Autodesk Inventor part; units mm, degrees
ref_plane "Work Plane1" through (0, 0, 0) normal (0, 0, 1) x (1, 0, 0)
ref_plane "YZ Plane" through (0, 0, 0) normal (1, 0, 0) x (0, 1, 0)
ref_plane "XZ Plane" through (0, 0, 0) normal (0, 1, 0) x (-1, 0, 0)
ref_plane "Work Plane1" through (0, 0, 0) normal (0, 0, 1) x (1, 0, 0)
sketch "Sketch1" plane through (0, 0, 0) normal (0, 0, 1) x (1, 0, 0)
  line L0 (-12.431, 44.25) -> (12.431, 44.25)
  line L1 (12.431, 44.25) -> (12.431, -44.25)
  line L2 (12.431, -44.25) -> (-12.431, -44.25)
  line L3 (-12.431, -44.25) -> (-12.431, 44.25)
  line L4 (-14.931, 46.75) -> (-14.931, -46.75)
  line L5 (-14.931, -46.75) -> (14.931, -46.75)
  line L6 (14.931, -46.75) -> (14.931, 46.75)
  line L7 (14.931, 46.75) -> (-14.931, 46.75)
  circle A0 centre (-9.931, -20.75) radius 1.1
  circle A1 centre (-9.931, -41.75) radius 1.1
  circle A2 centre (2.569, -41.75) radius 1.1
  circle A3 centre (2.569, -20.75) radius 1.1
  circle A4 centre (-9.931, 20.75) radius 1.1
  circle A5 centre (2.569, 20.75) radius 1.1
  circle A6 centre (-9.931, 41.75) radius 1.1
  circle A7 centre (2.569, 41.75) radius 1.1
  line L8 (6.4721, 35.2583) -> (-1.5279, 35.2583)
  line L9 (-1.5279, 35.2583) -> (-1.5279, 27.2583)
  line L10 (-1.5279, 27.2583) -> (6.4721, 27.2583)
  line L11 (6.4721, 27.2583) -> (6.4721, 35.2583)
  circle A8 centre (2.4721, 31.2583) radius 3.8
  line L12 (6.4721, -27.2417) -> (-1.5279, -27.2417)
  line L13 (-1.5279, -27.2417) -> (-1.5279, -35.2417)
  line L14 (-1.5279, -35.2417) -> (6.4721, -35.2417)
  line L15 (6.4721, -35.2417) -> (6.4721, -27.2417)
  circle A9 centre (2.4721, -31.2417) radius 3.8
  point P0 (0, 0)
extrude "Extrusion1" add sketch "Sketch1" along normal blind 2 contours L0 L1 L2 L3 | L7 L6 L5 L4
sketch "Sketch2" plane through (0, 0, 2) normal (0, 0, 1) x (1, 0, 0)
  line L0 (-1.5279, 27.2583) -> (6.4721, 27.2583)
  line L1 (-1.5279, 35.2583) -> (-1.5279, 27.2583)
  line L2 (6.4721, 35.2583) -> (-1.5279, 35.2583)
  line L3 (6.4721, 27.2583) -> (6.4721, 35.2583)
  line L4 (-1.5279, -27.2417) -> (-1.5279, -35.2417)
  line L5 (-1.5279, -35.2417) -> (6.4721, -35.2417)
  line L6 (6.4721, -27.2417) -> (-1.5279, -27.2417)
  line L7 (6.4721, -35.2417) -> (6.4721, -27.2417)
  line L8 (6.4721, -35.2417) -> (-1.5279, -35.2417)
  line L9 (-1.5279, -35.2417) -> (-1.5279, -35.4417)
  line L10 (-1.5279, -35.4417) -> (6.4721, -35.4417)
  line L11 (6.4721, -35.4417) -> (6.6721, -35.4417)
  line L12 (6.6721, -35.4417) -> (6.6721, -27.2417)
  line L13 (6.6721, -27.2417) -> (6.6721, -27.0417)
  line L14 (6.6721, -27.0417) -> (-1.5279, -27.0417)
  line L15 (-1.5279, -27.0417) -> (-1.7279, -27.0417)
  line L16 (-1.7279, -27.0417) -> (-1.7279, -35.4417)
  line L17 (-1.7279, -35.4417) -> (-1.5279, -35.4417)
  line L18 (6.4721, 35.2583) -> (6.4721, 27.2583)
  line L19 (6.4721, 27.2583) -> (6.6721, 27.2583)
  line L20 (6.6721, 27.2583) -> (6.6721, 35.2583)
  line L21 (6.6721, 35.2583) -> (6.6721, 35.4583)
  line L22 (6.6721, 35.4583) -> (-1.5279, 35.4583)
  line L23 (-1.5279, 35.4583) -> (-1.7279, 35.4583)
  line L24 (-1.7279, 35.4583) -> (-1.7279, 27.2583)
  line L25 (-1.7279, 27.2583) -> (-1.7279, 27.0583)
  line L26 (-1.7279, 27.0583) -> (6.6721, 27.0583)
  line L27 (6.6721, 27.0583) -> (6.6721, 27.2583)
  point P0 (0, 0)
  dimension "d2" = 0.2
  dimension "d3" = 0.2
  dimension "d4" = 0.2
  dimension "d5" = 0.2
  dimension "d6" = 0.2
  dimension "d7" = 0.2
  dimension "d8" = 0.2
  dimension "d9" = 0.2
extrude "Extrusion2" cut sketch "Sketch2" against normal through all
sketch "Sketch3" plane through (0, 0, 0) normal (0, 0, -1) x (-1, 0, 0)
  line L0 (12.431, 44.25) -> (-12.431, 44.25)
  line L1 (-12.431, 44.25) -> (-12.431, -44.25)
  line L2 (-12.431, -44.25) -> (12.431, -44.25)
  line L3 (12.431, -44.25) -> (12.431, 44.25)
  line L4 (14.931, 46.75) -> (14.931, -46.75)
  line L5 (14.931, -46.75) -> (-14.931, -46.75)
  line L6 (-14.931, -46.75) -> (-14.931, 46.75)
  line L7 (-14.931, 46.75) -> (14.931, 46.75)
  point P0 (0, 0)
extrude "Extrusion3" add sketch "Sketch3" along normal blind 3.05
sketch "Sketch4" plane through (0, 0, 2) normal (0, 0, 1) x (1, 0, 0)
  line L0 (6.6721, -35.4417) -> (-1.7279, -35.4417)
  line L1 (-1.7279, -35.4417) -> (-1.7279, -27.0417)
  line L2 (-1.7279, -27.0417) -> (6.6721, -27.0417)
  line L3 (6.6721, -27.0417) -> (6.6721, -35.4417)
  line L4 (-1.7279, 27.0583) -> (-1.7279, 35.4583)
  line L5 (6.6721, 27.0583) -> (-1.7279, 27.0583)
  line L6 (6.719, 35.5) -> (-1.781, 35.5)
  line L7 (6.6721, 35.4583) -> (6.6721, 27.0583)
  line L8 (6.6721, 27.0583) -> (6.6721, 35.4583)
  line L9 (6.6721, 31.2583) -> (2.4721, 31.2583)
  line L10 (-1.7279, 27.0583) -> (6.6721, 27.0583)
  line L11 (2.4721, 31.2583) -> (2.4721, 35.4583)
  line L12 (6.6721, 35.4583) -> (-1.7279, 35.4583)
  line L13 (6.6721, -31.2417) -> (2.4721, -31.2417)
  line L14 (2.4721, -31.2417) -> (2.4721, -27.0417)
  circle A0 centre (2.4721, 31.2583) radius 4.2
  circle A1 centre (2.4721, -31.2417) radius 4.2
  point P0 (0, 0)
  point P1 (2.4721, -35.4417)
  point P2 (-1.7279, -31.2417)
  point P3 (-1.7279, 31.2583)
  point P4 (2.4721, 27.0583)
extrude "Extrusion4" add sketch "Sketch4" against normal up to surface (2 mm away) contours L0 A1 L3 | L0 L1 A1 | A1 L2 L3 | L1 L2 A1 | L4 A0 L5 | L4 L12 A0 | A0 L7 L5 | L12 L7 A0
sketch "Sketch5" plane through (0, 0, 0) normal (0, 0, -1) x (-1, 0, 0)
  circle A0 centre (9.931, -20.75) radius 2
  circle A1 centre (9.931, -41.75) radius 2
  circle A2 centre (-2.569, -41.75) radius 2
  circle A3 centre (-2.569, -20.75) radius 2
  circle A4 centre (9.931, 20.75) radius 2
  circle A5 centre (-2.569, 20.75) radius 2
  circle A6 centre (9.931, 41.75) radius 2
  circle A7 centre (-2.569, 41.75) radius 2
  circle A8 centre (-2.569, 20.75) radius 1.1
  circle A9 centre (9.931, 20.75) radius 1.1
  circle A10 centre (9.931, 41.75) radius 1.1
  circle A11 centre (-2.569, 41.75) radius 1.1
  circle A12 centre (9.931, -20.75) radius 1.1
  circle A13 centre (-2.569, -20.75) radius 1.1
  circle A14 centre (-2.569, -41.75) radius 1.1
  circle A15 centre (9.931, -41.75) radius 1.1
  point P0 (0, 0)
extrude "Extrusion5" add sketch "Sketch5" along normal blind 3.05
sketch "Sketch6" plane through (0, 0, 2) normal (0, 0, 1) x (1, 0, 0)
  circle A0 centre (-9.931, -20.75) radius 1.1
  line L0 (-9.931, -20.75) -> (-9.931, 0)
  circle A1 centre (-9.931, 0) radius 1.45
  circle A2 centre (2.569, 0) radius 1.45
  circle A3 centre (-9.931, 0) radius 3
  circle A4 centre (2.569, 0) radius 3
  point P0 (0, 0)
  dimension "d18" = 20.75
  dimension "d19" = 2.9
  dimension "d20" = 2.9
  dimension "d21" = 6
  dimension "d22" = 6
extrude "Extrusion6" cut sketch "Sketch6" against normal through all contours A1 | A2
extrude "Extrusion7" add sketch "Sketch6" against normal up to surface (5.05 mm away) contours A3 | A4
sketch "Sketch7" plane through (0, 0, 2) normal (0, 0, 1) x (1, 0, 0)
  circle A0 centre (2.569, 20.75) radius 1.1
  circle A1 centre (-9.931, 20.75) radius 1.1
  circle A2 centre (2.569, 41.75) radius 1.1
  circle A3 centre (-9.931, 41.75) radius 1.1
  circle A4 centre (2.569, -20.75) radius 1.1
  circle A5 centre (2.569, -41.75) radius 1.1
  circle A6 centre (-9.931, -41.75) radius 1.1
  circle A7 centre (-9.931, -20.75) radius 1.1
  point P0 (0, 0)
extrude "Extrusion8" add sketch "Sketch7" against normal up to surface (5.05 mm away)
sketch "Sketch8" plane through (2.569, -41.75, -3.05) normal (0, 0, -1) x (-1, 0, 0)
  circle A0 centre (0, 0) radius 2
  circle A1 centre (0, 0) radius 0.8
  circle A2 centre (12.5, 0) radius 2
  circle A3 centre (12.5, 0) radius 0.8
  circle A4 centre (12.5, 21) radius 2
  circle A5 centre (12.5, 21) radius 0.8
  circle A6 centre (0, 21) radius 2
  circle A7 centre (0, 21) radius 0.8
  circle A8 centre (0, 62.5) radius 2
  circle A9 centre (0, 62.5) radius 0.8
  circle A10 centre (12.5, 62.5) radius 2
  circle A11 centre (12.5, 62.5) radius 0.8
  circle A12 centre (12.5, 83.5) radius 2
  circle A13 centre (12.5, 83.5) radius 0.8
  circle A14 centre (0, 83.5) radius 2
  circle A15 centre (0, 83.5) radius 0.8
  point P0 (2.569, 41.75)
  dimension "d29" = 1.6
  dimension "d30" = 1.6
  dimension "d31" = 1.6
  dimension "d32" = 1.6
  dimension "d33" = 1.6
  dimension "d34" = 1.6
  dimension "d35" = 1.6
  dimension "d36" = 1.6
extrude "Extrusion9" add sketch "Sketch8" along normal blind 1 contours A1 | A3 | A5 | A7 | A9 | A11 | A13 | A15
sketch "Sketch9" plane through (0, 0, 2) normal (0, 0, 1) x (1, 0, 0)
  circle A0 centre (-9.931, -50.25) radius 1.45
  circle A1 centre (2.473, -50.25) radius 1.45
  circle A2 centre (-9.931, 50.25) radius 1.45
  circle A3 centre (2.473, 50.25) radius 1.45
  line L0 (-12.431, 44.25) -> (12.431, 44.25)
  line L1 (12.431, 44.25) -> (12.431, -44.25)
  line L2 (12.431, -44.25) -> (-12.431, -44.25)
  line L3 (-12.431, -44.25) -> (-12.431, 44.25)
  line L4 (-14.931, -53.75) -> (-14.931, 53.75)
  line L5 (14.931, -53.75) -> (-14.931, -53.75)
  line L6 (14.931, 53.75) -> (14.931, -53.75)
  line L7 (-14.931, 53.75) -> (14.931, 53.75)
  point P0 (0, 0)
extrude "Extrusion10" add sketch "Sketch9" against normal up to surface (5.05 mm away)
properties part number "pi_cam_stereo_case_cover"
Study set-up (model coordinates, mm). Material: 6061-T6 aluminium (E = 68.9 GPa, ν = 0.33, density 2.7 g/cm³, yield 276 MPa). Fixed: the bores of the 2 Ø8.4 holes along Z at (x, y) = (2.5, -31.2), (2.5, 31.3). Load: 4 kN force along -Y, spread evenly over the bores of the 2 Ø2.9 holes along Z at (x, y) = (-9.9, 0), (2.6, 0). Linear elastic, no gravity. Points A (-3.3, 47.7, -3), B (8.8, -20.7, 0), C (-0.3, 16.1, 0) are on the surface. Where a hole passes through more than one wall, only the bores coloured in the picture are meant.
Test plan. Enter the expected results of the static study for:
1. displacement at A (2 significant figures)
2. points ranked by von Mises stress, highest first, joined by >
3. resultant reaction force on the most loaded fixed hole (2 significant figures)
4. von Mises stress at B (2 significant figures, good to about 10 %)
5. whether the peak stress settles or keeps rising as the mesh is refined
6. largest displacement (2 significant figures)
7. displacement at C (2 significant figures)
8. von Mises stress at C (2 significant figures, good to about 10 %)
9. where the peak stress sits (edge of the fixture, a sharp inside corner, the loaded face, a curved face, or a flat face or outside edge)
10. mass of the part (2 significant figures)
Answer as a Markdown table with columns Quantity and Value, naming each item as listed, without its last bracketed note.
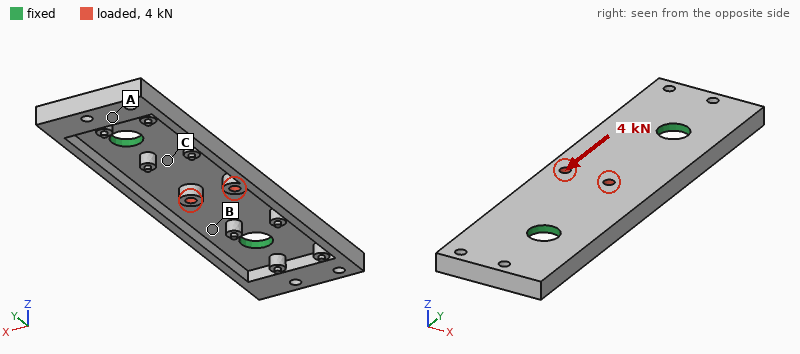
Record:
| Quantity | Value |
|---|---|
| displacement at A | 11 µm |
| points ranked by von Mises stress, highest first, joined by > | C > B > A |
| resultant reaction force on the most loaded fixed hole | 2.0 kN |
| von Mises stress at B | 27 MPa |
| whether the peak stress settles or keeps rising as the mesh is refined | keeps rising |
| largest displacement | 61 µm |
| displacement at C | 22 µm |
| von Mises stress at C | 50 MPa |
| where the peak stress sits | a sharp inside corner |
| mass of the part | 26 g |
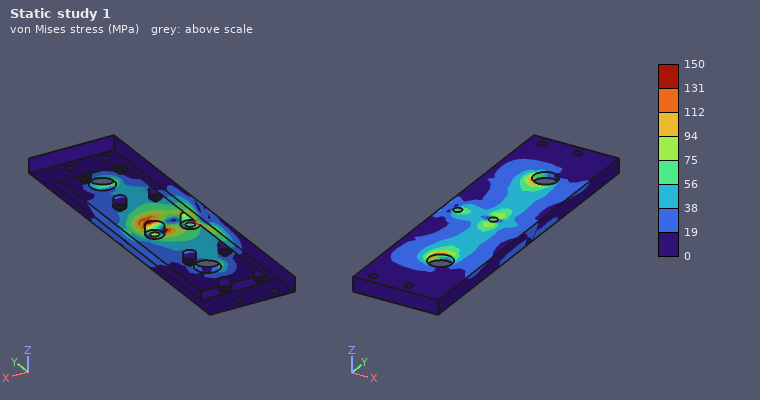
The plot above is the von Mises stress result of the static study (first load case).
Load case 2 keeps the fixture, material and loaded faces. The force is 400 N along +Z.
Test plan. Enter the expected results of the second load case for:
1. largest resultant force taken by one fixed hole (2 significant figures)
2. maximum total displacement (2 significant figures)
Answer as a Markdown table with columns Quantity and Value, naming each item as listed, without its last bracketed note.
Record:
| Quantity | Value |
|---|---|
| largest resultant force taken by one fixed hole | 290 N |
| maximum total displacement | 0.19 mm |
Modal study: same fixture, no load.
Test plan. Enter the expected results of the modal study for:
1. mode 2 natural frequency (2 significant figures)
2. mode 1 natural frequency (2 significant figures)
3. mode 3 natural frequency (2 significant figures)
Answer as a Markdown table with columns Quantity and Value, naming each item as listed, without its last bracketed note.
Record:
| Quantity | Value |
|---|---|
| mode 2 natural frequency | 3800 Hz |
| mode 1 natural frequency | 3300 Hz |
| mode 3 natural frequency | 3800 Hz |
